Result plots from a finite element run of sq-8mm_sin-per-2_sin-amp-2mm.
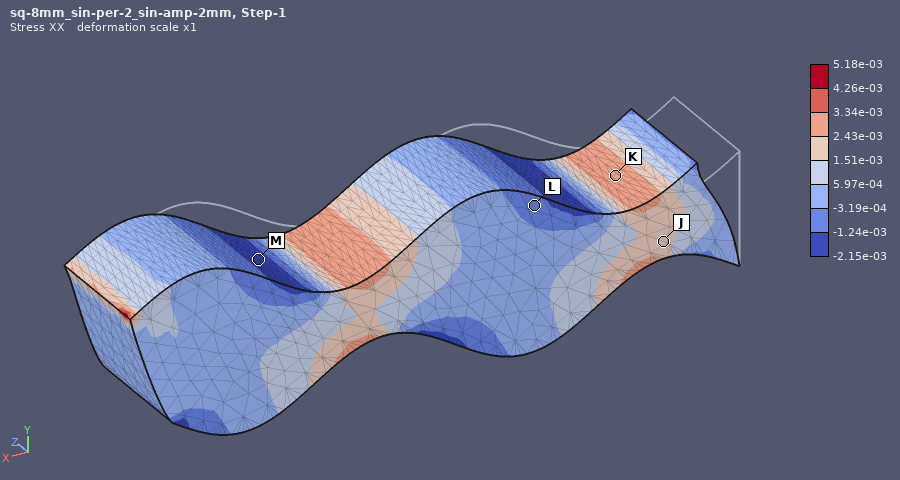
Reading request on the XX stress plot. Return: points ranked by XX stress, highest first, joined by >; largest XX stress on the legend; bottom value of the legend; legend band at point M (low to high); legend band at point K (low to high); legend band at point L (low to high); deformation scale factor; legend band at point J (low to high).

K > J > L > M
5.18e-03
-2.15e-03
-2.15e-03 to -1.24e-03
2.43e-03 to 3.34e-03
-1.24e-03 to -3.19e-04
1
1.51e-03 to 2.43e-03
